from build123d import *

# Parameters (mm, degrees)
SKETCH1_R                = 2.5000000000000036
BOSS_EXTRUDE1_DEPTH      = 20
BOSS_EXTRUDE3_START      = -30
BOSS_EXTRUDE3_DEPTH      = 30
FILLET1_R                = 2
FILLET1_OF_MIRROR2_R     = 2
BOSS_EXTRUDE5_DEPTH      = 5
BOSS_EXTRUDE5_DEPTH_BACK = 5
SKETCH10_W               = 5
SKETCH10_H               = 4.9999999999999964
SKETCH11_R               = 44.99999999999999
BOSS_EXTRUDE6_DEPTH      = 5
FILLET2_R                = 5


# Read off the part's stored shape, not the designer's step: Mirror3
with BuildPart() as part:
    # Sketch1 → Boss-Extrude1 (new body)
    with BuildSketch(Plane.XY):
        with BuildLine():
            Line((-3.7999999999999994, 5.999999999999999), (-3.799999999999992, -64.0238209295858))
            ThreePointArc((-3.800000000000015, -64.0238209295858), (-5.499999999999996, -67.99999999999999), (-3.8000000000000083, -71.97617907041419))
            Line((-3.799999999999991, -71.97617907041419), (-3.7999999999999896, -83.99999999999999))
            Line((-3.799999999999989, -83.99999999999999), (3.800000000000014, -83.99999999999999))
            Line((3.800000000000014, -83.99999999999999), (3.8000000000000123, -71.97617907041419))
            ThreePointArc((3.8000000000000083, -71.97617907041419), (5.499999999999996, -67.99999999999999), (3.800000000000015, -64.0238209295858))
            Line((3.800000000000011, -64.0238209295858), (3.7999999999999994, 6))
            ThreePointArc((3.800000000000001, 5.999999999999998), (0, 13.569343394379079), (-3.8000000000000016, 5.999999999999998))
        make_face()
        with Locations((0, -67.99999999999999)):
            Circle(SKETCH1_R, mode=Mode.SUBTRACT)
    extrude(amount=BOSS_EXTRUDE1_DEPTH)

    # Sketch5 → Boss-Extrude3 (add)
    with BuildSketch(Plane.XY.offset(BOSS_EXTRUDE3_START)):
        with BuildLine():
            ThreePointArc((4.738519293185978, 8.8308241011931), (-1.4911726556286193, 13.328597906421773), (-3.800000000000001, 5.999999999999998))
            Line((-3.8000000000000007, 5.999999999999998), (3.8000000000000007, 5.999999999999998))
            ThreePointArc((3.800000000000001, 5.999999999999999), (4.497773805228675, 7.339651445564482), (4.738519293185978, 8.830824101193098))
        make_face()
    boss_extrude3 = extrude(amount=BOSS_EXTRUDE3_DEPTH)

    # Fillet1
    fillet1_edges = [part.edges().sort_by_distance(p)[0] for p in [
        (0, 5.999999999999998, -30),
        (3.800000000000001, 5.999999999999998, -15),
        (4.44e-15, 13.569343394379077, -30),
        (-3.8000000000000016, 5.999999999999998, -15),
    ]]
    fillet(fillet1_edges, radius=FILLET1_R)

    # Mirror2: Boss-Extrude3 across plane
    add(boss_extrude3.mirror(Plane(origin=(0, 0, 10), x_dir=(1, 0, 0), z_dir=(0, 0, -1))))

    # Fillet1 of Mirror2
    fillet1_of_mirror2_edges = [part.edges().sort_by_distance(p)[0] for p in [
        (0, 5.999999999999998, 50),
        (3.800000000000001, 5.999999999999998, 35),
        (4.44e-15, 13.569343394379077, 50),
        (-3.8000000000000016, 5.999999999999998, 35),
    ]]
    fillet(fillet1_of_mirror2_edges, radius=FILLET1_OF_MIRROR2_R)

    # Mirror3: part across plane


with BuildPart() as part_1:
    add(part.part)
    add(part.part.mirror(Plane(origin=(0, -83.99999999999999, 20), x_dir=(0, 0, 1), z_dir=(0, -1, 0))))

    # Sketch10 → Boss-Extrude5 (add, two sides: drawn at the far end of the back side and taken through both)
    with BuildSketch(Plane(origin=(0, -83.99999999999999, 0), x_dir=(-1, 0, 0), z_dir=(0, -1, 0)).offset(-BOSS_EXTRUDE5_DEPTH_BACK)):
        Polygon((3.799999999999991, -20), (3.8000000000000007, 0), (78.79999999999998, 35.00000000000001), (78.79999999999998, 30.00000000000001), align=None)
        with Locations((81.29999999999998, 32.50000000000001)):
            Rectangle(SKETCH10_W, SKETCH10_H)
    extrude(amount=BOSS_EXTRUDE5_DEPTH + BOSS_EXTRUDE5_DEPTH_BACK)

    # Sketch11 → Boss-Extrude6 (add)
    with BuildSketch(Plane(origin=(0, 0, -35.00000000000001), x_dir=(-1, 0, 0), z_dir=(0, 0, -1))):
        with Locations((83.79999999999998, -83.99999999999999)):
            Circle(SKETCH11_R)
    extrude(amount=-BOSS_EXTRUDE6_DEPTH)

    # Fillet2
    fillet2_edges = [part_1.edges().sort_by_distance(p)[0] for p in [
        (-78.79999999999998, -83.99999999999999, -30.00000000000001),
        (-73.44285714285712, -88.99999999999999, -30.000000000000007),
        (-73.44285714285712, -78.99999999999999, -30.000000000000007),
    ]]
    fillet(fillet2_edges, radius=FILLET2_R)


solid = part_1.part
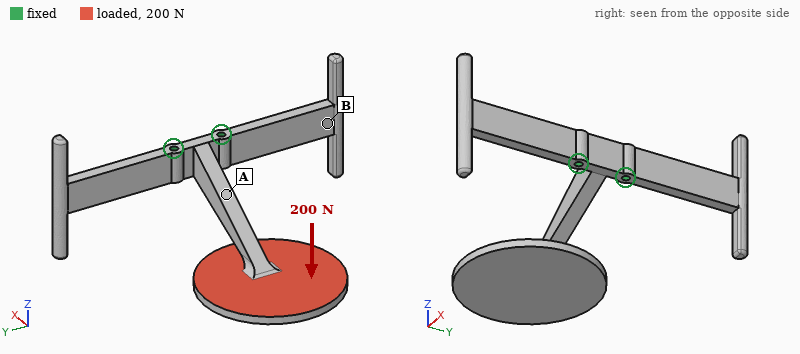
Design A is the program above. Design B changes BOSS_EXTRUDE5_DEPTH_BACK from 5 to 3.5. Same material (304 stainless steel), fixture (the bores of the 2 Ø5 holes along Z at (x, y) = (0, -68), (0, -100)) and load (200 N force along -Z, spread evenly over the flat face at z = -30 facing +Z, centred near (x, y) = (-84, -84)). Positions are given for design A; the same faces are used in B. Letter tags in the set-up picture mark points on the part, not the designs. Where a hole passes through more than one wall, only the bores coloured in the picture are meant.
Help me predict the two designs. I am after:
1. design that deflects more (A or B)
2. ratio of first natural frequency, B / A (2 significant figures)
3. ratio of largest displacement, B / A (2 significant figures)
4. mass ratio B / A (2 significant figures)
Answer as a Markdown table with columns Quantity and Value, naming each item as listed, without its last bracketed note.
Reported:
| Quantity | Value |
|---|---|
| design that deflects more | B |
| ratio of first natural frequency, B / A | 0.80 |
| ratio of largest displacement, B / A | 1.2 |
| mass ratio B / A | 0.98 |
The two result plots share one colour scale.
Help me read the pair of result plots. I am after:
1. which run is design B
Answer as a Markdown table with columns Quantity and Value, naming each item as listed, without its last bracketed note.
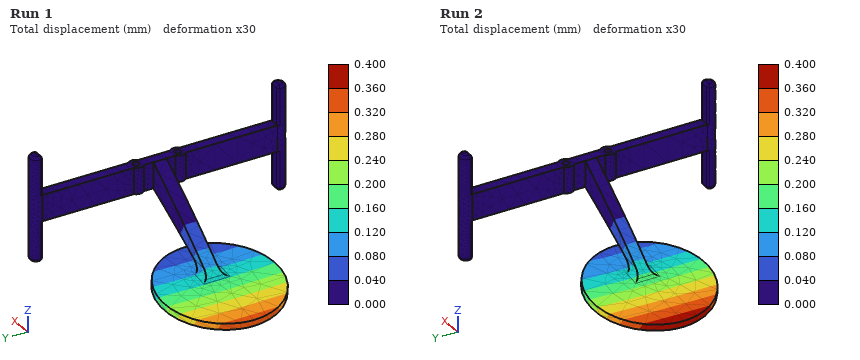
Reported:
| Quantity | Value |
|---|---|
| which run is design B | Run 2 |
